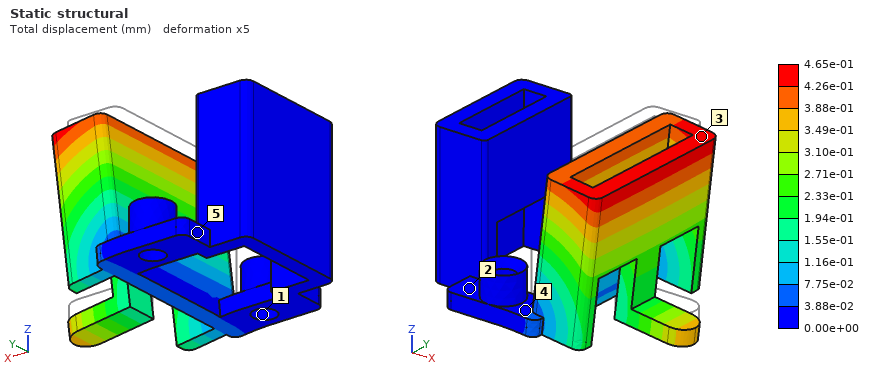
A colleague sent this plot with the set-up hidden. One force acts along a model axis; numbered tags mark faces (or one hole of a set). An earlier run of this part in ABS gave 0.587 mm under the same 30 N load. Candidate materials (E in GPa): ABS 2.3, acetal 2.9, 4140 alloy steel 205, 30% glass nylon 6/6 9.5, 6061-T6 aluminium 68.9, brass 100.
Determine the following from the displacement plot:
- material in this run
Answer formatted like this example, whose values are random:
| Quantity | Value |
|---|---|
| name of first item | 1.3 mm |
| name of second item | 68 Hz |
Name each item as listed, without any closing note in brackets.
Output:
| Quantity | Value |
|---|---|
| material in this run | acetal |
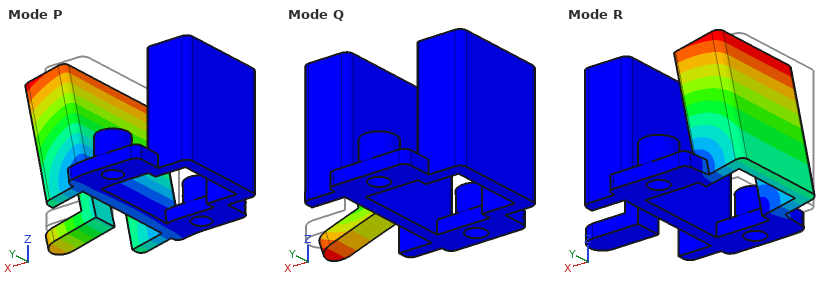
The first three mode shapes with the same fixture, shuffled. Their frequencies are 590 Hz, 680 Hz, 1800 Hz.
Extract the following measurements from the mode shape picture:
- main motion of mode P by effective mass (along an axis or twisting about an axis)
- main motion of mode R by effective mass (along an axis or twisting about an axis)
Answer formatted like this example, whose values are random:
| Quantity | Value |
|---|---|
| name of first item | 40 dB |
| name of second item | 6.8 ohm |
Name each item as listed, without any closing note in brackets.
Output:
| Quantity | Value |
|---|---|
| main motion of mode P by effective mass | along X |
| main motion of mode R by effective mass | along X |
